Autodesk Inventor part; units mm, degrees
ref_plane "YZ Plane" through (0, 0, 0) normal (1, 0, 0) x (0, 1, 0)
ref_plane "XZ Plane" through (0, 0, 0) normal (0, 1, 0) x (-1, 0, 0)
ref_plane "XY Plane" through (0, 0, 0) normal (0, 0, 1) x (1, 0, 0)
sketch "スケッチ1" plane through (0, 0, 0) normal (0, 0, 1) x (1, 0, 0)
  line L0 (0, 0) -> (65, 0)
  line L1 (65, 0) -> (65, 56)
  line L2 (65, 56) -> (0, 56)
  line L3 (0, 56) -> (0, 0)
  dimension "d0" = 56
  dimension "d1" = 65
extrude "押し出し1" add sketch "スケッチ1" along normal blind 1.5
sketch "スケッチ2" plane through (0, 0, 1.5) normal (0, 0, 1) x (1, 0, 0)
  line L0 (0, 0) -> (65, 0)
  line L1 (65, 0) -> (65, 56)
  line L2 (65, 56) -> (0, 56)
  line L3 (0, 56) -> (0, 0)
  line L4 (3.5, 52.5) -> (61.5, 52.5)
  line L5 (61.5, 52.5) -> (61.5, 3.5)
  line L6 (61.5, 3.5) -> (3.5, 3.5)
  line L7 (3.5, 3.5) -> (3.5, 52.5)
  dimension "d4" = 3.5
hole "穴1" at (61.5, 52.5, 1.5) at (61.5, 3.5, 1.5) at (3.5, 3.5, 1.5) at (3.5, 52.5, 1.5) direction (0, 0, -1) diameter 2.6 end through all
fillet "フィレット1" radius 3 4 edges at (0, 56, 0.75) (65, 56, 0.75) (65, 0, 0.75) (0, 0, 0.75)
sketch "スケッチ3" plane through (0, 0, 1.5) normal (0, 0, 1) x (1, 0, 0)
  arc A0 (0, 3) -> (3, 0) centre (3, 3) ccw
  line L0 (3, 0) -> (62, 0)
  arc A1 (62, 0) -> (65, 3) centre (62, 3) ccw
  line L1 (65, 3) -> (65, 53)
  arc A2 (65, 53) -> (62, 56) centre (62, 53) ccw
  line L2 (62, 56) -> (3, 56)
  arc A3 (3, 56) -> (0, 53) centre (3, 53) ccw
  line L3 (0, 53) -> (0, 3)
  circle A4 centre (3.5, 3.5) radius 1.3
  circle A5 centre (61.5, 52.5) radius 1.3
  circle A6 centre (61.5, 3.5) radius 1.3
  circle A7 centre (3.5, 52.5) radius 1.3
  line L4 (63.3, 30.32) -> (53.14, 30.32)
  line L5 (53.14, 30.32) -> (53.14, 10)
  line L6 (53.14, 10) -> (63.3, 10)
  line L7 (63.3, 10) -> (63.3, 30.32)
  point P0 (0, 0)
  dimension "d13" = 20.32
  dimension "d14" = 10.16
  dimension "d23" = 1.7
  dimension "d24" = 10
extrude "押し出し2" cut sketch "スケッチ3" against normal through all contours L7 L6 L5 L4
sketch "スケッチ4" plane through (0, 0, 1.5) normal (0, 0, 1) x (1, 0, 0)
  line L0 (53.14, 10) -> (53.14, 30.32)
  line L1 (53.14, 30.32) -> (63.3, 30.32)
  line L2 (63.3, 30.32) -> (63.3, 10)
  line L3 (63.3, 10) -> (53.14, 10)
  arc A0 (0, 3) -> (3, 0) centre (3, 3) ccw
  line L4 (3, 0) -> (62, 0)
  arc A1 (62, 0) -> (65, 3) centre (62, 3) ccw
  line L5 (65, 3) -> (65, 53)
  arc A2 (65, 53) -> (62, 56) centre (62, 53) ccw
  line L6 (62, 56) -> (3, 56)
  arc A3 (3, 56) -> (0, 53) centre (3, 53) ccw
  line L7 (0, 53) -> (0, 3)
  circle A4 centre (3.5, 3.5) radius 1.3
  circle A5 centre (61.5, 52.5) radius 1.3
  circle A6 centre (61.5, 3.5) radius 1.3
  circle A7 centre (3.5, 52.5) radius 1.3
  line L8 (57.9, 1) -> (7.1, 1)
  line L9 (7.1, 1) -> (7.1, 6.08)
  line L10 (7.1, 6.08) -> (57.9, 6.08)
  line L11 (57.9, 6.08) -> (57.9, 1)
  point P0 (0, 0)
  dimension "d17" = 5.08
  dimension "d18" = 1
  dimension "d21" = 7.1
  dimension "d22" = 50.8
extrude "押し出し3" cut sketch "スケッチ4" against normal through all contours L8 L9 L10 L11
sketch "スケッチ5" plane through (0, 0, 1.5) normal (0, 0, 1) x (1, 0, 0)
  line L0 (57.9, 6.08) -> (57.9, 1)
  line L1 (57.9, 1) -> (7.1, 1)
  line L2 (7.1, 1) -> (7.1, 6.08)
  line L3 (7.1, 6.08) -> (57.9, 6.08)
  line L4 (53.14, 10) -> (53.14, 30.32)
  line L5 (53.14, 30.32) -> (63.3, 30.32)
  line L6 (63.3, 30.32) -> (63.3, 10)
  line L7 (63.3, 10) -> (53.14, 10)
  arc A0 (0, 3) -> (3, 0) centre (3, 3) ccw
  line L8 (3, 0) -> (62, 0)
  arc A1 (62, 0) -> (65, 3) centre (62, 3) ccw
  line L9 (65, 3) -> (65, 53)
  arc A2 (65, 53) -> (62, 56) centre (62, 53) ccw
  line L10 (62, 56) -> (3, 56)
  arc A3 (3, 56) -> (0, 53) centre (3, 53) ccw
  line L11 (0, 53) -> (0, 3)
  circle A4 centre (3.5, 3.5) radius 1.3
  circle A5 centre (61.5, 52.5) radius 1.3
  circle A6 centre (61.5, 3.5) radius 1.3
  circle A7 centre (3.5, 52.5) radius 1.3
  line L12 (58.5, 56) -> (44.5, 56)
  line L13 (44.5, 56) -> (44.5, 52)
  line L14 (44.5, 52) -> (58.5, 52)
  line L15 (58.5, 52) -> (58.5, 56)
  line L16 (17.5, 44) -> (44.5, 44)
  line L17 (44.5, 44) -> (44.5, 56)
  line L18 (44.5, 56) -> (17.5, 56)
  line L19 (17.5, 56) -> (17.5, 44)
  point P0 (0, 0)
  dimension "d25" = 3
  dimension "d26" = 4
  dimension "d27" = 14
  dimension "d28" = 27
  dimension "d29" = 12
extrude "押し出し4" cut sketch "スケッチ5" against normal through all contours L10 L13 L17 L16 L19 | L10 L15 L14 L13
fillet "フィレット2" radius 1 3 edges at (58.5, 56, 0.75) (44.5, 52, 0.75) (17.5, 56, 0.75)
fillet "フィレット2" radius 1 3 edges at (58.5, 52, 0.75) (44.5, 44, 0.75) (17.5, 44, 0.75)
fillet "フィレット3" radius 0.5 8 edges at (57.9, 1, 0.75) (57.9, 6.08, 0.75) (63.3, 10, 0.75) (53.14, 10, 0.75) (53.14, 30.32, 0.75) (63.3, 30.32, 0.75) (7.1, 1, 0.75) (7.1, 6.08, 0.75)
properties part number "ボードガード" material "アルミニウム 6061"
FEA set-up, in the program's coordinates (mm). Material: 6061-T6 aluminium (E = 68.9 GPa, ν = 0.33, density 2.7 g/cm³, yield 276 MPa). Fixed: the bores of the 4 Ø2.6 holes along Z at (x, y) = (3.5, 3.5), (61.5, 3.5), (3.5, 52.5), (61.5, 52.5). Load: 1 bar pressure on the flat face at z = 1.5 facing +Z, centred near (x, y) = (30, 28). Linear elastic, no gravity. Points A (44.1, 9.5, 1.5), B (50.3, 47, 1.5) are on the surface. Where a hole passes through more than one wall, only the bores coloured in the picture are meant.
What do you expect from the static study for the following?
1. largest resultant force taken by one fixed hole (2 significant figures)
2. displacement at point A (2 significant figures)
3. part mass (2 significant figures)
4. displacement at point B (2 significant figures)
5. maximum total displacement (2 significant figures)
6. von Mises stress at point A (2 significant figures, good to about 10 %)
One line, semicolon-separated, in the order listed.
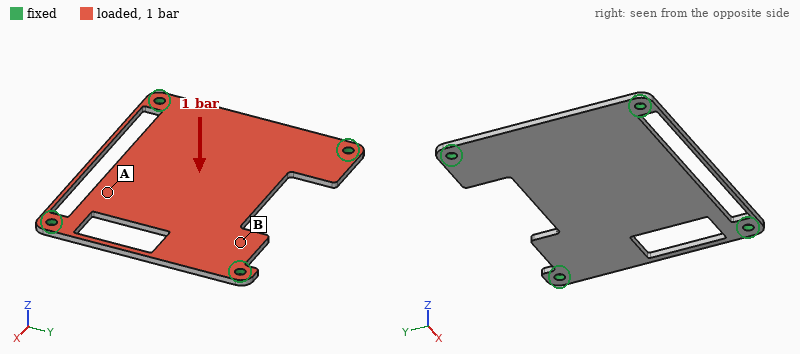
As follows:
76 N; 0.25 mm; 11 g; 0.14 mm; 0.35 mm; 49 MPa
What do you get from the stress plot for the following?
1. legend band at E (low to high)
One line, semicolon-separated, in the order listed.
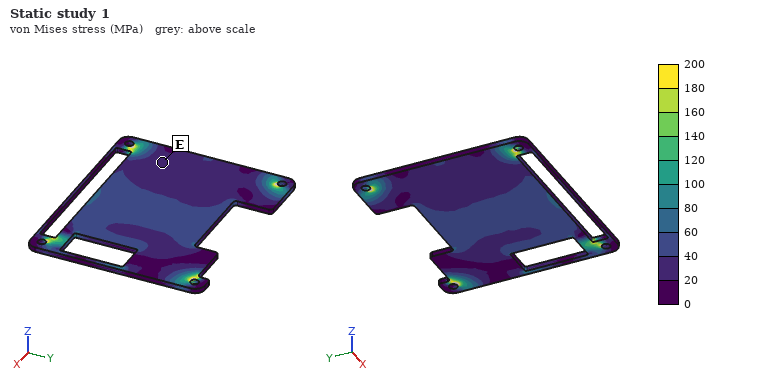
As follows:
20 to 40 MPa
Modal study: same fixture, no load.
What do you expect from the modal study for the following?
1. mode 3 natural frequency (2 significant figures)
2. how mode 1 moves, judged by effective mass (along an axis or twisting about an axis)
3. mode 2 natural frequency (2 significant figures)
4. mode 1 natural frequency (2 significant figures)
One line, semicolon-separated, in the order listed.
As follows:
2700 Hz; along Z; 2000 Hz; 1500 Hz
